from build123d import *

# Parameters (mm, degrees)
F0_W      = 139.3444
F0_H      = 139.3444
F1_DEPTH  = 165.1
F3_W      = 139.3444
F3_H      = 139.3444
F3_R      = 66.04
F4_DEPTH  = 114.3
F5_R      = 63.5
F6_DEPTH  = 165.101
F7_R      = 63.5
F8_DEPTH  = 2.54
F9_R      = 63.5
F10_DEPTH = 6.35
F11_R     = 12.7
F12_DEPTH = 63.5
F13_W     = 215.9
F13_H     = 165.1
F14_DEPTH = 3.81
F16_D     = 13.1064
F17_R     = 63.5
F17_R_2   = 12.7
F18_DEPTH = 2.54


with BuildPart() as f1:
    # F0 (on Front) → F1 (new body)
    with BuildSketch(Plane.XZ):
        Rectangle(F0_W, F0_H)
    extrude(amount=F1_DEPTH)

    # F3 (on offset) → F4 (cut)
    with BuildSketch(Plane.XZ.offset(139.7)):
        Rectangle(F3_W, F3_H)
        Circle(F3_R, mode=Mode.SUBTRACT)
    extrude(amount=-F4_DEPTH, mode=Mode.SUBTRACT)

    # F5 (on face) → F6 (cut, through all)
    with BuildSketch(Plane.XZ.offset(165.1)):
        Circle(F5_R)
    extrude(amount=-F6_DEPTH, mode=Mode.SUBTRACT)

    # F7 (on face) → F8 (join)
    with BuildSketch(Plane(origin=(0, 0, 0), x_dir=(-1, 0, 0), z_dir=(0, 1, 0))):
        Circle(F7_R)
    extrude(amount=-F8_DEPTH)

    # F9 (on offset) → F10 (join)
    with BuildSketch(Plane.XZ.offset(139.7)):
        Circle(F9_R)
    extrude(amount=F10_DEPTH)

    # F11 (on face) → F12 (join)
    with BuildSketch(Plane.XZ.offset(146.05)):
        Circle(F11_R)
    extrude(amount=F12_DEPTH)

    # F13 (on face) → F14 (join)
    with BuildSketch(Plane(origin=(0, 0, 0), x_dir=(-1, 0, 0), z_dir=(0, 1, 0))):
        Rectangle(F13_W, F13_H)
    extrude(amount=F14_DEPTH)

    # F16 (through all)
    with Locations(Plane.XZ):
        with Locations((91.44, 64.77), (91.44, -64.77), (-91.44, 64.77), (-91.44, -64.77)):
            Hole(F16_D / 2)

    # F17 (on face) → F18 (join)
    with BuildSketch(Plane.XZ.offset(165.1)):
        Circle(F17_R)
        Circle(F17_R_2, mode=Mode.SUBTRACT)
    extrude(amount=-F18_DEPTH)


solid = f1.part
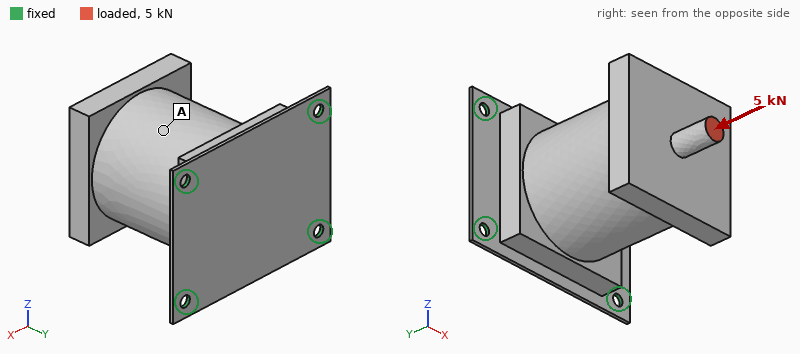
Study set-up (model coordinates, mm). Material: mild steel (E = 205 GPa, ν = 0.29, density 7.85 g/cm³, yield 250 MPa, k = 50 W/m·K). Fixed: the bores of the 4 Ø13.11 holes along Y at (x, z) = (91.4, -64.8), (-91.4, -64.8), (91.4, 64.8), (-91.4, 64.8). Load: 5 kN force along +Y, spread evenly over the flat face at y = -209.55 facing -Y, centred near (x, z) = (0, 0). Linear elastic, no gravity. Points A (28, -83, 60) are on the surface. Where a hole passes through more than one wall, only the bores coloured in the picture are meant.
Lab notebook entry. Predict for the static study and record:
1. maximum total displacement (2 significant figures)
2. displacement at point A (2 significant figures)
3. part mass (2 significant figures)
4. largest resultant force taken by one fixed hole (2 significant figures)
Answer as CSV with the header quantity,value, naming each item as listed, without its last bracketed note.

quantity,value
maximum total displacement,94 µm
displacement at point A,32 µm
part mass,6.0 kg
largest resultant force taken by one fixed hole,1.7 kN
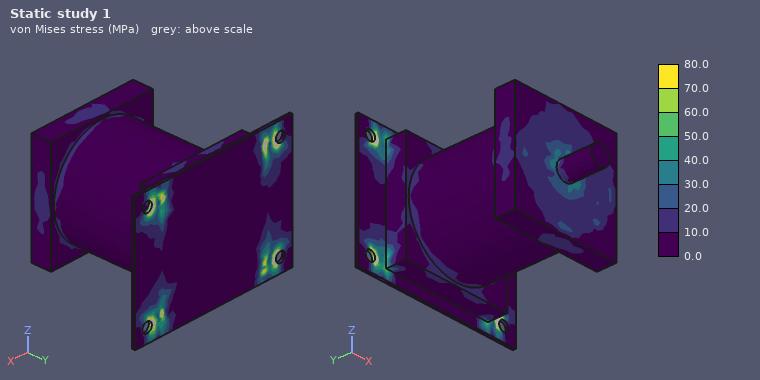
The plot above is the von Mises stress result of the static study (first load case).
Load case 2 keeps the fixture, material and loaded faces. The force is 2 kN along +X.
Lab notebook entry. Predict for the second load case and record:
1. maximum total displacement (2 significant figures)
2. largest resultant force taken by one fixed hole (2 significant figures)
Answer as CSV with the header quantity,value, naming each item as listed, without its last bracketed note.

quantity,value
maximum total displacement,0.16 mm
largest resultant force taken by one fixed hole,1.5 kN
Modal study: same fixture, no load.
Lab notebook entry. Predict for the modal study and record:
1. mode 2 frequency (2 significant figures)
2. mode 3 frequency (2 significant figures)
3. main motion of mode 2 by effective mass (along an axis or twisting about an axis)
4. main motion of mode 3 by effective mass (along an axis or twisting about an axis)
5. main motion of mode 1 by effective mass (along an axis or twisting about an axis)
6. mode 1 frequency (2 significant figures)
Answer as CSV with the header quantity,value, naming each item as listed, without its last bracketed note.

quantity,value
mode 2 frequency,520 Hz
mode 3 frequency,830 Hz
main motion of mode 2 by effective mass,along X
main motion of mode 3 by effective mass,along Y
main motion of mode 1 by effective mass,along Z
mode 1 frequency,410 Hz
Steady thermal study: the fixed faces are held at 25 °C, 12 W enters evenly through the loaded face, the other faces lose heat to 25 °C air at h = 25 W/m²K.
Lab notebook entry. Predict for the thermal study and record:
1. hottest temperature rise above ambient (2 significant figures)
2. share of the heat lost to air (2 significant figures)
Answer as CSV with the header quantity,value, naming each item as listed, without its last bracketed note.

quantity,value
hottest temperature rise above ambient,30 K
share of the heat lost to air,99 %
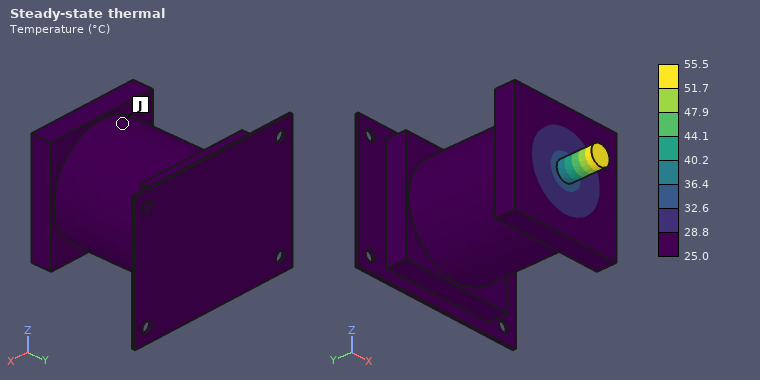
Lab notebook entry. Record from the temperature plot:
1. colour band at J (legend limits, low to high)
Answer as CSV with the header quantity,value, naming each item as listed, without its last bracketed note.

quantity,value
colour band at J,25.0 to 28.8 °C
